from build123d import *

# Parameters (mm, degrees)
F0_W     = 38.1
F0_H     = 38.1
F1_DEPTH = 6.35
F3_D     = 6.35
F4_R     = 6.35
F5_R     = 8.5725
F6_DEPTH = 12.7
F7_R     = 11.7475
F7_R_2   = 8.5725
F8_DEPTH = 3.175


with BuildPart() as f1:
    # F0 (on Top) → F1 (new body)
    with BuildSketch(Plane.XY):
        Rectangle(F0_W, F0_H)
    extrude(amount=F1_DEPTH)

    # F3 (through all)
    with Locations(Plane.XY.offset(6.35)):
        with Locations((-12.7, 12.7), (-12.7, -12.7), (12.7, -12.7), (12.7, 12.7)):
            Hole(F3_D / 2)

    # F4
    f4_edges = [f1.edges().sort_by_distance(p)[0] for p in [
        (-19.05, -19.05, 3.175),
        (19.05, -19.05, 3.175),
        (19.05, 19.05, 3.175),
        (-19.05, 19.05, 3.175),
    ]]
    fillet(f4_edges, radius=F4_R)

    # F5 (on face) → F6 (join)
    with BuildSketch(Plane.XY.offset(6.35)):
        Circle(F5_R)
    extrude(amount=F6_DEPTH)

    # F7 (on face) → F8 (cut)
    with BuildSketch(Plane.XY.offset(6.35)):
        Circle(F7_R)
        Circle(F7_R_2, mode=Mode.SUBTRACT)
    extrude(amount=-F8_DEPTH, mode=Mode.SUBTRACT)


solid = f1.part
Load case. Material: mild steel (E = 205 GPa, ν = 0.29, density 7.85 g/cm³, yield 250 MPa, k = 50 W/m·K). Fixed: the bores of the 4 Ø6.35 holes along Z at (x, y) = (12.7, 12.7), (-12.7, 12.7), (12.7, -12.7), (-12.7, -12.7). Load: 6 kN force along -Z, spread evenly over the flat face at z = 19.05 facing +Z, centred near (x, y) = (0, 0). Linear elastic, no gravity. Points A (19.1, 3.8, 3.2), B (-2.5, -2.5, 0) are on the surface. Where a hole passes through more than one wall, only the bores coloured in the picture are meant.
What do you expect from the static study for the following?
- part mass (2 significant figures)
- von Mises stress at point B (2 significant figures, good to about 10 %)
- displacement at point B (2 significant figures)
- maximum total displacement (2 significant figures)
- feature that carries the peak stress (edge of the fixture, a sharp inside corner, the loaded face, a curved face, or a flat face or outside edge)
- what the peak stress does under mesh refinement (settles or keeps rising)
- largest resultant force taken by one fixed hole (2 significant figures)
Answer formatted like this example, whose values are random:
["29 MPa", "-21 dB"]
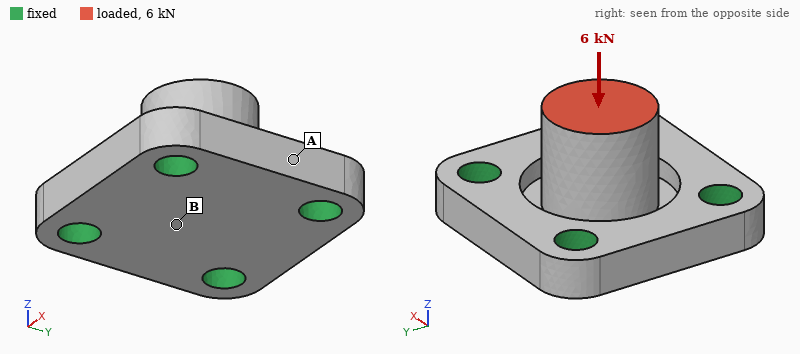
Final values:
["82 g", "50 MPa", "8.9 µm", "10 µm", "edge of the fixture", "keeps rising", "1.5 kN"]
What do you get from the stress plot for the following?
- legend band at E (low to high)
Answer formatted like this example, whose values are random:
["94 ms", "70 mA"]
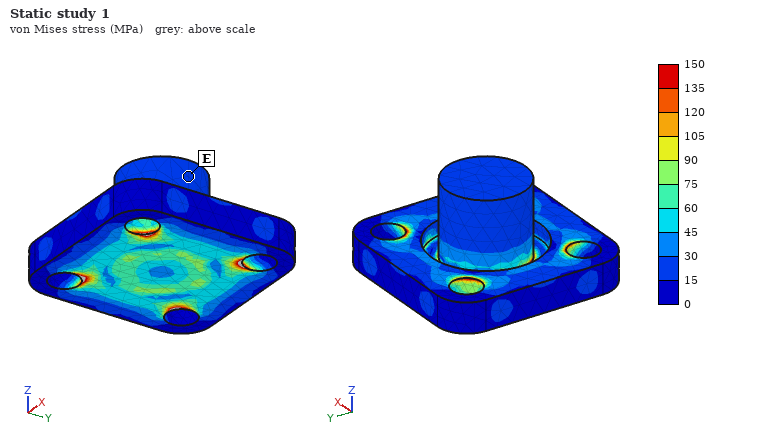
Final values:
["15 to 30 MPa"]
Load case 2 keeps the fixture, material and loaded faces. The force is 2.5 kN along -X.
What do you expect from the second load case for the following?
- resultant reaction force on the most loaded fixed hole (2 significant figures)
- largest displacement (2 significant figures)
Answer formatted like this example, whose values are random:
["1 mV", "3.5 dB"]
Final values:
["1.3 kN", "26 µm"]
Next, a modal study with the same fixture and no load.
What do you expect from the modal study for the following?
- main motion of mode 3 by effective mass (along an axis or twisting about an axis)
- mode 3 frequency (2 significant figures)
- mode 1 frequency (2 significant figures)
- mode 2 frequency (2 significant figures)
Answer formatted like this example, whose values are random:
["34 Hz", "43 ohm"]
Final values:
["along Z", "21 kHz", "15 kHz", "15 kHz"]
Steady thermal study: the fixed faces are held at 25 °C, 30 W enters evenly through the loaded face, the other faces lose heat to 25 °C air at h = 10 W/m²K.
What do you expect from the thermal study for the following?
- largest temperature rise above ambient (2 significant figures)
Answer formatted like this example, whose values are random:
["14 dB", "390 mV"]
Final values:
["67 K"]
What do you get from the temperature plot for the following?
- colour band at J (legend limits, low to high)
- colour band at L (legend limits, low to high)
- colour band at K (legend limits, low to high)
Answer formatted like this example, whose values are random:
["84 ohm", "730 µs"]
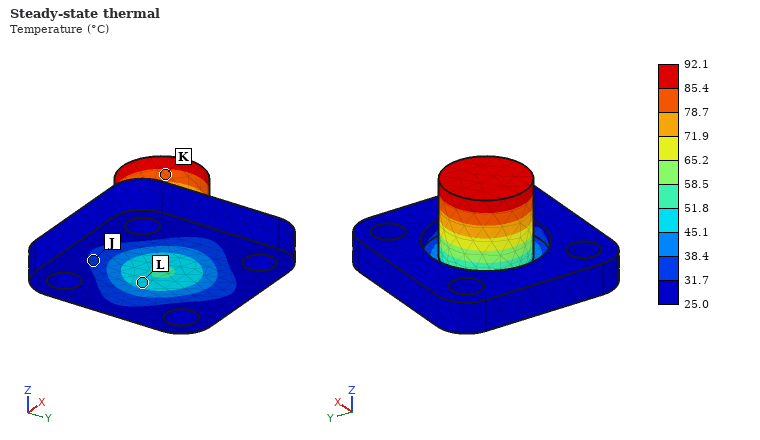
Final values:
["31.7 to 38.4 °C", "45.1 to 51.8 °C", "78.7 to 85.4 °C"]
